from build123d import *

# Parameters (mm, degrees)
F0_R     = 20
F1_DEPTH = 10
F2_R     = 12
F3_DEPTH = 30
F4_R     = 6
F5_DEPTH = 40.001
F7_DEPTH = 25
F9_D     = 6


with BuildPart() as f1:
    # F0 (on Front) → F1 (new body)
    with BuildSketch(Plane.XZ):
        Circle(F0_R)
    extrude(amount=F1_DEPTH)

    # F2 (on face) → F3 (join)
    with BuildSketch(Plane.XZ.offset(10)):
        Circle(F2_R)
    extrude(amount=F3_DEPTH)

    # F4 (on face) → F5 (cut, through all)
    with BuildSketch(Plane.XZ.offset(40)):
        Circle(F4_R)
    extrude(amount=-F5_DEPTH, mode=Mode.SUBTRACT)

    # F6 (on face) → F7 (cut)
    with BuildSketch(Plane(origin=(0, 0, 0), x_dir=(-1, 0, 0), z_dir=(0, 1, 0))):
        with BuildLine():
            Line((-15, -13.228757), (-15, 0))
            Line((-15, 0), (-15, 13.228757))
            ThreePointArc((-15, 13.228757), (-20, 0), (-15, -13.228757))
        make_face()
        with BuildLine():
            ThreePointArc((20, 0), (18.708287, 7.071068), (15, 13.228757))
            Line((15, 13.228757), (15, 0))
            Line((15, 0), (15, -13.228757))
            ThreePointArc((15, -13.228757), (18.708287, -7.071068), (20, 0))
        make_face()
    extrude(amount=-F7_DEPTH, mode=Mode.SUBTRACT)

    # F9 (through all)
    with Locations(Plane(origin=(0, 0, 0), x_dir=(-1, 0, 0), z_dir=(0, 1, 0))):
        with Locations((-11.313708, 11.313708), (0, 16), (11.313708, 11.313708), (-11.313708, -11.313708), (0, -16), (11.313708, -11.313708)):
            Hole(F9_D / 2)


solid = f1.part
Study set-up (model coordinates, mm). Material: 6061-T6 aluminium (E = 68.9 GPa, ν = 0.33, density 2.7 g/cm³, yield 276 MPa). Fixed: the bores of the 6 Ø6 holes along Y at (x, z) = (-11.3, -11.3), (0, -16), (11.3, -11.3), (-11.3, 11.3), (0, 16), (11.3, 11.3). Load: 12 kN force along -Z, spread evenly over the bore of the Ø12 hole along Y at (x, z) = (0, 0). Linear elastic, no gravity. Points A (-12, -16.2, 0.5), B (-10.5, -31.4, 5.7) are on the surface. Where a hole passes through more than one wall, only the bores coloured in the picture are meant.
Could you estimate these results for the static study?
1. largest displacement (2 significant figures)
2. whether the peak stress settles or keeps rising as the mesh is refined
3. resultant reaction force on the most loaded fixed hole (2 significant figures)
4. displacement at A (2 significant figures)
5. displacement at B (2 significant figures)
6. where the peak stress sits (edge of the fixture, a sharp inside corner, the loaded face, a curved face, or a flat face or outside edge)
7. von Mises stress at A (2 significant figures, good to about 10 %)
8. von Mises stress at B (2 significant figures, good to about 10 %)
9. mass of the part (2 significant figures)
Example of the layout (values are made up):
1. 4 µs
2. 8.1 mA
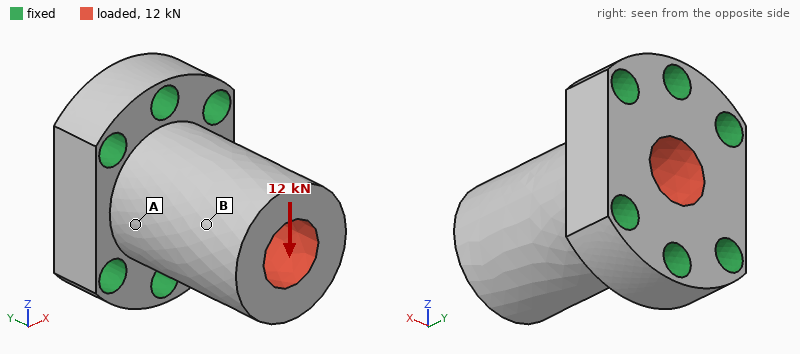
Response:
1. 73 µm
2. keeps rising
3. 4.1 kN
4. 14 µm
5. 52 µm
6. edge of the fixture
7. 43 MPa
8. 19 MPa
9. 49 g
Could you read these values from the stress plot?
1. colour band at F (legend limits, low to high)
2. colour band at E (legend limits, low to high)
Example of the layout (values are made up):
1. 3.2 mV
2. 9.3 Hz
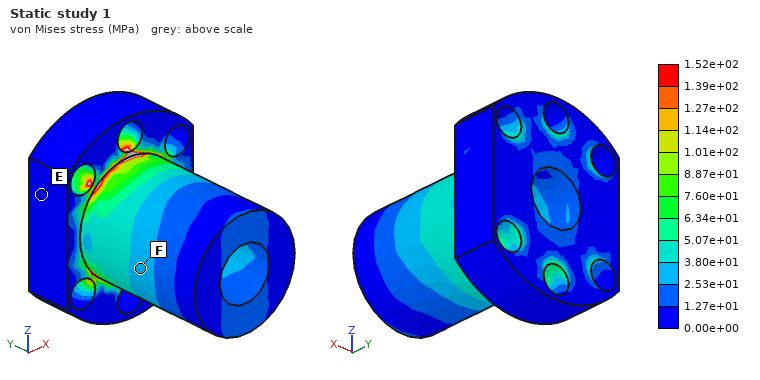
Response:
1. 2.53e+01 to 3.80e+01 MPa
2. 0.00e+00 to 1.27e+01 MPa
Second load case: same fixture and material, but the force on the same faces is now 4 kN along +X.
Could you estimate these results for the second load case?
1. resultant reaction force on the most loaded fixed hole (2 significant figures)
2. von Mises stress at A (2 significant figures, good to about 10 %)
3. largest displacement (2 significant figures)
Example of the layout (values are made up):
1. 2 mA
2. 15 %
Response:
1. 1.6 kN
2. 21 MPa
3. 29 µm
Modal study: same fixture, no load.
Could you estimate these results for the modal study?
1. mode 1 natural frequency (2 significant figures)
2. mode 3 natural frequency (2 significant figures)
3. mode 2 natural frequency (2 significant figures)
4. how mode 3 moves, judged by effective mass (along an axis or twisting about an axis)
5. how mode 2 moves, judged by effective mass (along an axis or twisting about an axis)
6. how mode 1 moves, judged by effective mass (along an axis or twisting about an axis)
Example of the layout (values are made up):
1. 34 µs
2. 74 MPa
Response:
1. 12 kHz
2. 24 kHz
3. 13 kHz
4. twisting about Y
5. along Z
6. along X
